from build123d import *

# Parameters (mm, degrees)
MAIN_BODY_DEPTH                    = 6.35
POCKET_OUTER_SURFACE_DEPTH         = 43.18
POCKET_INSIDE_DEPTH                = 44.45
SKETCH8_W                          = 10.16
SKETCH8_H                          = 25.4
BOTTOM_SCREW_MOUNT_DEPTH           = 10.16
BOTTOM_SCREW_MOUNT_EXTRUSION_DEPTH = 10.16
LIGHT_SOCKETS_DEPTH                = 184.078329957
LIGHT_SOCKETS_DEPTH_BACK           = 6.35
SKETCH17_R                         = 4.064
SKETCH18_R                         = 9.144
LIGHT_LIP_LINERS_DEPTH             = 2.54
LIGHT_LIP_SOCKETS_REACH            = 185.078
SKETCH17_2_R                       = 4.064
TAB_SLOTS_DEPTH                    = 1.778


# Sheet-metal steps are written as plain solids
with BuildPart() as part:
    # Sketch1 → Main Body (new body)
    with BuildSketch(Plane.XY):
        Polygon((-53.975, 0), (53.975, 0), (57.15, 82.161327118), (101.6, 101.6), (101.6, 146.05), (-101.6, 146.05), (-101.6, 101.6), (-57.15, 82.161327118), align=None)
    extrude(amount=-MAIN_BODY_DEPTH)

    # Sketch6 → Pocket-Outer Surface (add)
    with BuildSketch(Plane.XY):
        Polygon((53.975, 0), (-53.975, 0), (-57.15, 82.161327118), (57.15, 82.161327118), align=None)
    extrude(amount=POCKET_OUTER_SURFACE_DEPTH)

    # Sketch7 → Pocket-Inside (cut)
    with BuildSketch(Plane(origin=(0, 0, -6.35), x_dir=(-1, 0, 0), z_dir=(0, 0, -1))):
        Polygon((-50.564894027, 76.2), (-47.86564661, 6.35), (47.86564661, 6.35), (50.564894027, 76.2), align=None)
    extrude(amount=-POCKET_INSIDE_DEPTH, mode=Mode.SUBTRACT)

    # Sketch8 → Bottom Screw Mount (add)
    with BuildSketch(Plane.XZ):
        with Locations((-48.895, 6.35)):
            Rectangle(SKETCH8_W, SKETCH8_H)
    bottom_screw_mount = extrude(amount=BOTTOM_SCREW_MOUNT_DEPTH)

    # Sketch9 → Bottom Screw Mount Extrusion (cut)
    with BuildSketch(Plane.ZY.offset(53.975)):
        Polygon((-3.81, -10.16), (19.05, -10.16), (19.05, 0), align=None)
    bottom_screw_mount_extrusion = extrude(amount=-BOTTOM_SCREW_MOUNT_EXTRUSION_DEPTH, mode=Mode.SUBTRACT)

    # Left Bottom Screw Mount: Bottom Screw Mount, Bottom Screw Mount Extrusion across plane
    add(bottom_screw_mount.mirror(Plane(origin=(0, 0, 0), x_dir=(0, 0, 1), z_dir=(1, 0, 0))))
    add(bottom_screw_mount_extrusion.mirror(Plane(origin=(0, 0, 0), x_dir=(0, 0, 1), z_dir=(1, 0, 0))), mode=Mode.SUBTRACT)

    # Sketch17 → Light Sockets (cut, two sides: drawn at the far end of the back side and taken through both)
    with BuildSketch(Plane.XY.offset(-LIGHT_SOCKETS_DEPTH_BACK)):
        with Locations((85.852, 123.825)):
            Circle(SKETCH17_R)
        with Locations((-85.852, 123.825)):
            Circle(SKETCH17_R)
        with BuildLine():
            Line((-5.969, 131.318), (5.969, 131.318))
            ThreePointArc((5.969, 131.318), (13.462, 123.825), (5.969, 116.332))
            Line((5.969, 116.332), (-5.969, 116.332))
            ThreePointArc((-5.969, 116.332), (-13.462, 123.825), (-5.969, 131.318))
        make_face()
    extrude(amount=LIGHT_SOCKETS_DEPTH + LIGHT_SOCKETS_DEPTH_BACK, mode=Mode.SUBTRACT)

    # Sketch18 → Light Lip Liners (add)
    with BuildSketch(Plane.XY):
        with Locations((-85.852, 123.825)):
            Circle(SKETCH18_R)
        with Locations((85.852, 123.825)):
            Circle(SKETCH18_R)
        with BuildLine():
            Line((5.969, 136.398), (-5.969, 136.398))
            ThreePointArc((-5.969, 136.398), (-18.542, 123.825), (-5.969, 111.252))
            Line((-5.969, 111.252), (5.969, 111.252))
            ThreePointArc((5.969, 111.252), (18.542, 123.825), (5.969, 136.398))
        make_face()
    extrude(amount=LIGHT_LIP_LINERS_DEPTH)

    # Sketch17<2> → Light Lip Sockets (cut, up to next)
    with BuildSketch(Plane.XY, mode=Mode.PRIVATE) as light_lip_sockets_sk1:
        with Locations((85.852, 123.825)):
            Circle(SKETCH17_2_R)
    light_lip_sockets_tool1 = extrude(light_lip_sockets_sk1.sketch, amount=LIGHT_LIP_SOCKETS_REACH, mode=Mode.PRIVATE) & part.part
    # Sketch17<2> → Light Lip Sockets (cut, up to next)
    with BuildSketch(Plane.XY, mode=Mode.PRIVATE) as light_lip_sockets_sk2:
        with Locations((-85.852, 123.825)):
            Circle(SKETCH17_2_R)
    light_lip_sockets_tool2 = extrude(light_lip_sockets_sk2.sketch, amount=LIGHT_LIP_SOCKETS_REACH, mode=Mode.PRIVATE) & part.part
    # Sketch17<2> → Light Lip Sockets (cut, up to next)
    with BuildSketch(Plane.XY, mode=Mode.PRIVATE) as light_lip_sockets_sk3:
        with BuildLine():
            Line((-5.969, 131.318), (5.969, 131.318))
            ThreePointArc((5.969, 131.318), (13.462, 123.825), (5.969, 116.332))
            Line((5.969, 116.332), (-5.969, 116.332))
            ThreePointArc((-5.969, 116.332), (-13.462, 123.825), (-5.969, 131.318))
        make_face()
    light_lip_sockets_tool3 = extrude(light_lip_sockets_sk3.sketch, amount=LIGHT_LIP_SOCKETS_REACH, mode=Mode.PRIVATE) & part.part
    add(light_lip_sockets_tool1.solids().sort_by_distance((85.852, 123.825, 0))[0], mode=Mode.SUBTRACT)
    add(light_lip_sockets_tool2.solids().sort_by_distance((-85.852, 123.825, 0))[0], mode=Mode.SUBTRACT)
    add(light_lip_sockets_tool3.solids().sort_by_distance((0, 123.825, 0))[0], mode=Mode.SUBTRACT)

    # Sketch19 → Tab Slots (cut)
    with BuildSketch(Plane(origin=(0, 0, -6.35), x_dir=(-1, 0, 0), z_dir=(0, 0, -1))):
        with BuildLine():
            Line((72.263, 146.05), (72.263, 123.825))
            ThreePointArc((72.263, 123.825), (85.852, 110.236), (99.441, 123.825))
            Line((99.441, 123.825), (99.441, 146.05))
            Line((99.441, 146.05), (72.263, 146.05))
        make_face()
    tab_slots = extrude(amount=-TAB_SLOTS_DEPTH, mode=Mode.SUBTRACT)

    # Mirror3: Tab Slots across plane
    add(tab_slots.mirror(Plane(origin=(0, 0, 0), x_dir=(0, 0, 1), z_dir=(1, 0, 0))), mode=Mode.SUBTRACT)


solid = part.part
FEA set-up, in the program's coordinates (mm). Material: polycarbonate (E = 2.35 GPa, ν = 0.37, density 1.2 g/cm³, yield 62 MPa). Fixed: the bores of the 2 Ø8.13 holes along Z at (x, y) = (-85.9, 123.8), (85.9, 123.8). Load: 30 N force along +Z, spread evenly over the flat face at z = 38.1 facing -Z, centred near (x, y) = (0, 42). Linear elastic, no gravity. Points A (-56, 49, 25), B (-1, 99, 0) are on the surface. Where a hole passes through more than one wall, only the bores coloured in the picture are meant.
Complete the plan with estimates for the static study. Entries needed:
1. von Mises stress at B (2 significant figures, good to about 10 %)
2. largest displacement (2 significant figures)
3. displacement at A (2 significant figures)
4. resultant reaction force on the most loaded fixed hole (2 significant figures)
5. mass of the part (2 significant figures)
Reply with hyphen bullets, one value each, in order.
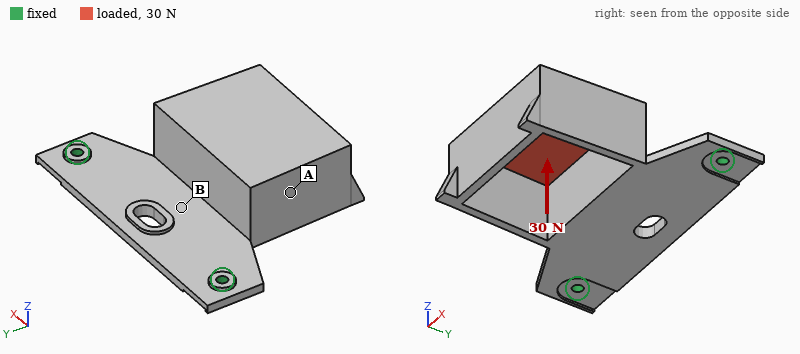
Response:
- 0.95 MPa
- 2.4 mm
- 1.4 mm
- 16 N
- 270 g
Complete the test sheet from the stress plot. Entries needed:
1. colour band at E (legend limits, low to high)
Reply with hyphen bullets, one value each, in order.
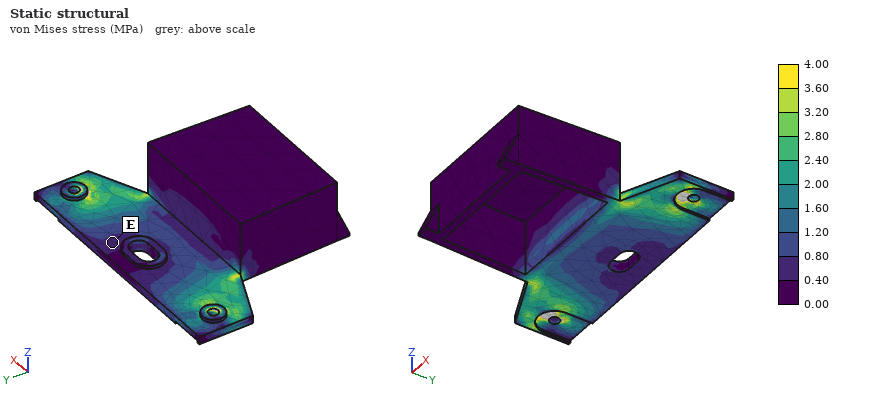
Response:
- 0.40 to 0.80 MPa
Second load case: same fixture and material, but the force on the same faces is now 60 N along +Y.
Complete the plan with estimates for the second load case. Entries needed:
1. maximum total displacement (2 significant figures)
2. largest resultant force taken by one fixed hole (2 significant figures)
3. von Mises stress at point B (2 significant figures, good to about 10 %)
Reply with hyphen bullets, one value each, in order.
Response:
- 3.0 mm
- 32 N
- 1.6 MPa
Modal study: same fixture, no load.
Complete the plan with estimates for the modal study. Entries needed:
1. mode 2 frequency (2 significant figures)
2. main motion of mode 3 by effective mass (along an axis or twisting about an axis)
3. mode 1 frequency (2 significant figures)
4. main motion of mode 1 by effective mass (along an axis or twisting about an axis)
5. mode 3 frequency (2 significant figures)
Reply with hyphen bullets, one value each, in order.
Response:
- 180 Hz
- along X
- 46 Hz
- along Z
- 240 Hz
